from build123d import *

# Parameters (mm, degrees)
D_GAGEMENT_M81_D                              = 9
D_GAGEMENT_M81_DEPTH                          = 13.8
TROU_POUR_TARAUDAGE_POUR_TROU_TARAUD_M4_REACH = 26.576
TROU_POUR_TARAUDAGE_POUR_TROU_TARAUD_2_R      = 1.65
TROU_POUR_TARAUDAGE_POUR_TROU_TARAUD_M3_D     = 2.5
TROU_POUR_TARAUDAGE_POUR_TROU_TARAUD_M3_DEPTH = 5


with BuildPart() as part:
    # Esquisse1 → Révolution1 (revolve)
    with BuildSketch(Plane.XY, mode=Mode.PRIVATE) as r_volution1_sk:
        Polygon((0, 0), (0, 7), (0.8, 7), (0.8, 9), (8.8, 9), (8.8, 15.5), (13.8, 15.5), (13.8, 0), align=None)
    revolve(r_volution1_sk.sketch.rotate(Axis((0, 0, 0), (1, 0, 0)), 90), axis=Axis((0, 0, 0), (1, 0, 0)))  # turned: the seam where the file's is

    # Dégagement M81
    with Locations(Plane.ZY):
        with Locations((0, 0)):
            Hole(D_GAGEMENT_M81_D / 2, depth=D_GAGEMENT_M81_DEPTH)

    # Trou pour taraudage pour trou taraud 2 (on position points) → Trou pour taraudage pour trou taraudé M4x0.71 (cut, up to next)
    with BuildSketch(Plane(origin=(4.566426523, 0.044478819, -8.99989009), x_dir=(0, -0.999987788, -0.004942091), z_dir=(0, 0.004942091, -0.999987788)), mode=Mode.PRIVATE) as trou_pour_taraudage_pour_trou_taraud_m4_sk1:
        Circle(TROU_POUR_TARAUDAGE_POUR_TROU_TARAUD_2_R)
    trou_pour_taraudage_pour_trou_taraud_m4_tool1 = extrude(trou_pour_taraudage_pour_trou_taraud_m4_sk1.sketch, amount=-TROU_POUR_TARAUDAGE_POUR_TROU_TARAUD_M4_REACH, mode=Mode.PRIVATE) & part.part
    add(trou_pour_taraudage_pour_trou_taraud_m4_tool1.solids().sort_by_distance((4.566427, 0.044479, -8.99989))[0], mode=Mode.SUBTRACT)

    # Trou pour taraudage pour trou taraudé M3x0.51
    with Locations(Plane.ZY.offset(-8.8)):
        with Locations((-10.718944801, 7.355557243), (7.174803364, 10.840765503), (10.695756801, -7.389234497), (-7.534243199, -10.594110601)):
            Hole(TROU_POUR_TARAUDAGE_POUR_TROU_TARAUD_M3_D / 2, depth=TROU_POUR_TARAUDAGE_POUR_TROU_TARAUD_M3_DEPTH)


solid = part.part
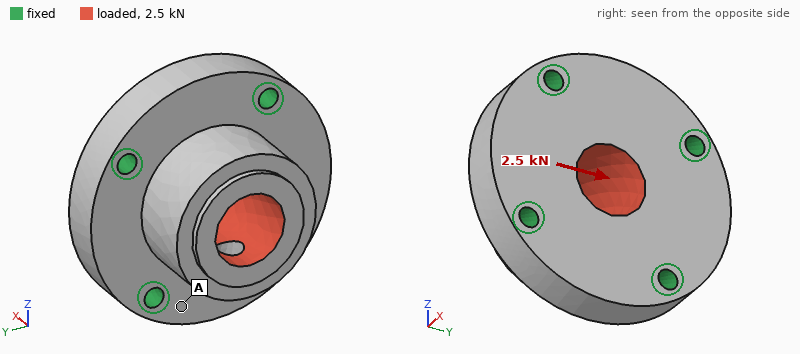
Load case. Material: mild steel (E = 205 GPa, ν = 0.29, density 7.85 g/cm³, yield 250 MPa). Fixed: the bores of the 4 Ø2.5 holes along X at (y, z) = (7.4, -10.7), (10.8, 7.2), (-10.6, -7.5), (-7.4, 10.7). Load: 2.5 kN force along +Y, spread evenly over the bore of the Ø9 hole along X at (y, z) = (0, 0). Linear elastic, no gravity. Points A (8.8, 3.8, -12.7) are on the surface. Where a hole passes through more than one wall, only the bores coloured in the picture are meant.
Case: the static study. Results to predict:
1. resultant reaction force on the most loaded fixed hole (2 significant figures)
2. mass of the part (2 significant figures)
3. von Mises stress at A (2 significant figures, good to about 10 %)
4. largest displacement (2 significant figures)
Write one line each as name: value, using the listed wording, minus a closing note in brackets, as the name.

resultant reaction force on the most loaded fixed hole: 790 N
mass of the part: 39 g
von Mises stress at A: 7.4 MPa
largest displacement: 2.9 µm
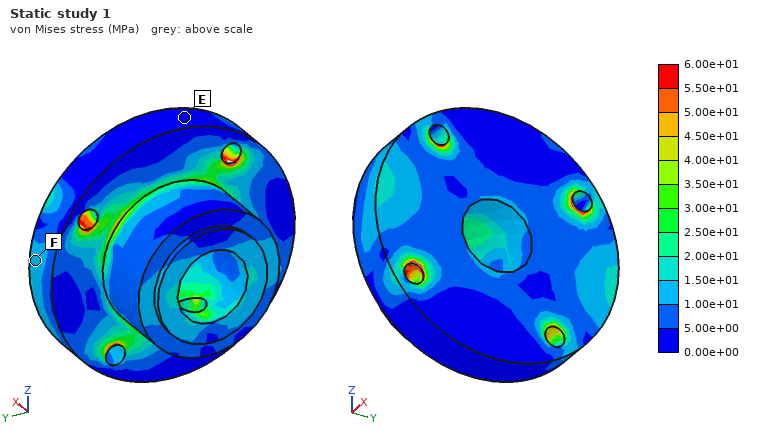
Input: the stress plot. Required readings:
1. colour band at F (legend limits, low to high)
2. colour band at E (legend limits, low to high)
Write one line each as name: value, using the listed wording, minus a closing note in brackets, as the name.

colour band at F: 1.00e+01 to 1.50e+01 MPa
colour band at E: 0.00e+00 to 5.00e+00 MPa
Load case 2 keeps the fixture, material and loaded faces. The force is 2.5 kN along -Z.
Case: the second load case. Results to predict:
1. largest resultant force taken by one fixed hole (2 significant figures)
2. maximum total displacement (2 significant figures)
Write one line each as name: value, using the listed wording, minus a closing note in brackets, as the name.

largest resultant force taken by one fixed hole: 780 N
maximum total displacement: 2.8 µm
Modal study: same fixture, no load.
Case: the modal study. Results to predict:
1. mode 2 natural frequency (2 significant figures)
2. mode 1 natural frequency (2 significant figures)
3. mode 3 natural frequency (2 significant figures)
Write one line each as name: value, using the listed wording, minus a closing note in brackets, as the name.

mode 2 natural frequency: 38 kHz
mode 1 natural frequency: 37 kHz
mode 3 natural frequency: 39 kHz
